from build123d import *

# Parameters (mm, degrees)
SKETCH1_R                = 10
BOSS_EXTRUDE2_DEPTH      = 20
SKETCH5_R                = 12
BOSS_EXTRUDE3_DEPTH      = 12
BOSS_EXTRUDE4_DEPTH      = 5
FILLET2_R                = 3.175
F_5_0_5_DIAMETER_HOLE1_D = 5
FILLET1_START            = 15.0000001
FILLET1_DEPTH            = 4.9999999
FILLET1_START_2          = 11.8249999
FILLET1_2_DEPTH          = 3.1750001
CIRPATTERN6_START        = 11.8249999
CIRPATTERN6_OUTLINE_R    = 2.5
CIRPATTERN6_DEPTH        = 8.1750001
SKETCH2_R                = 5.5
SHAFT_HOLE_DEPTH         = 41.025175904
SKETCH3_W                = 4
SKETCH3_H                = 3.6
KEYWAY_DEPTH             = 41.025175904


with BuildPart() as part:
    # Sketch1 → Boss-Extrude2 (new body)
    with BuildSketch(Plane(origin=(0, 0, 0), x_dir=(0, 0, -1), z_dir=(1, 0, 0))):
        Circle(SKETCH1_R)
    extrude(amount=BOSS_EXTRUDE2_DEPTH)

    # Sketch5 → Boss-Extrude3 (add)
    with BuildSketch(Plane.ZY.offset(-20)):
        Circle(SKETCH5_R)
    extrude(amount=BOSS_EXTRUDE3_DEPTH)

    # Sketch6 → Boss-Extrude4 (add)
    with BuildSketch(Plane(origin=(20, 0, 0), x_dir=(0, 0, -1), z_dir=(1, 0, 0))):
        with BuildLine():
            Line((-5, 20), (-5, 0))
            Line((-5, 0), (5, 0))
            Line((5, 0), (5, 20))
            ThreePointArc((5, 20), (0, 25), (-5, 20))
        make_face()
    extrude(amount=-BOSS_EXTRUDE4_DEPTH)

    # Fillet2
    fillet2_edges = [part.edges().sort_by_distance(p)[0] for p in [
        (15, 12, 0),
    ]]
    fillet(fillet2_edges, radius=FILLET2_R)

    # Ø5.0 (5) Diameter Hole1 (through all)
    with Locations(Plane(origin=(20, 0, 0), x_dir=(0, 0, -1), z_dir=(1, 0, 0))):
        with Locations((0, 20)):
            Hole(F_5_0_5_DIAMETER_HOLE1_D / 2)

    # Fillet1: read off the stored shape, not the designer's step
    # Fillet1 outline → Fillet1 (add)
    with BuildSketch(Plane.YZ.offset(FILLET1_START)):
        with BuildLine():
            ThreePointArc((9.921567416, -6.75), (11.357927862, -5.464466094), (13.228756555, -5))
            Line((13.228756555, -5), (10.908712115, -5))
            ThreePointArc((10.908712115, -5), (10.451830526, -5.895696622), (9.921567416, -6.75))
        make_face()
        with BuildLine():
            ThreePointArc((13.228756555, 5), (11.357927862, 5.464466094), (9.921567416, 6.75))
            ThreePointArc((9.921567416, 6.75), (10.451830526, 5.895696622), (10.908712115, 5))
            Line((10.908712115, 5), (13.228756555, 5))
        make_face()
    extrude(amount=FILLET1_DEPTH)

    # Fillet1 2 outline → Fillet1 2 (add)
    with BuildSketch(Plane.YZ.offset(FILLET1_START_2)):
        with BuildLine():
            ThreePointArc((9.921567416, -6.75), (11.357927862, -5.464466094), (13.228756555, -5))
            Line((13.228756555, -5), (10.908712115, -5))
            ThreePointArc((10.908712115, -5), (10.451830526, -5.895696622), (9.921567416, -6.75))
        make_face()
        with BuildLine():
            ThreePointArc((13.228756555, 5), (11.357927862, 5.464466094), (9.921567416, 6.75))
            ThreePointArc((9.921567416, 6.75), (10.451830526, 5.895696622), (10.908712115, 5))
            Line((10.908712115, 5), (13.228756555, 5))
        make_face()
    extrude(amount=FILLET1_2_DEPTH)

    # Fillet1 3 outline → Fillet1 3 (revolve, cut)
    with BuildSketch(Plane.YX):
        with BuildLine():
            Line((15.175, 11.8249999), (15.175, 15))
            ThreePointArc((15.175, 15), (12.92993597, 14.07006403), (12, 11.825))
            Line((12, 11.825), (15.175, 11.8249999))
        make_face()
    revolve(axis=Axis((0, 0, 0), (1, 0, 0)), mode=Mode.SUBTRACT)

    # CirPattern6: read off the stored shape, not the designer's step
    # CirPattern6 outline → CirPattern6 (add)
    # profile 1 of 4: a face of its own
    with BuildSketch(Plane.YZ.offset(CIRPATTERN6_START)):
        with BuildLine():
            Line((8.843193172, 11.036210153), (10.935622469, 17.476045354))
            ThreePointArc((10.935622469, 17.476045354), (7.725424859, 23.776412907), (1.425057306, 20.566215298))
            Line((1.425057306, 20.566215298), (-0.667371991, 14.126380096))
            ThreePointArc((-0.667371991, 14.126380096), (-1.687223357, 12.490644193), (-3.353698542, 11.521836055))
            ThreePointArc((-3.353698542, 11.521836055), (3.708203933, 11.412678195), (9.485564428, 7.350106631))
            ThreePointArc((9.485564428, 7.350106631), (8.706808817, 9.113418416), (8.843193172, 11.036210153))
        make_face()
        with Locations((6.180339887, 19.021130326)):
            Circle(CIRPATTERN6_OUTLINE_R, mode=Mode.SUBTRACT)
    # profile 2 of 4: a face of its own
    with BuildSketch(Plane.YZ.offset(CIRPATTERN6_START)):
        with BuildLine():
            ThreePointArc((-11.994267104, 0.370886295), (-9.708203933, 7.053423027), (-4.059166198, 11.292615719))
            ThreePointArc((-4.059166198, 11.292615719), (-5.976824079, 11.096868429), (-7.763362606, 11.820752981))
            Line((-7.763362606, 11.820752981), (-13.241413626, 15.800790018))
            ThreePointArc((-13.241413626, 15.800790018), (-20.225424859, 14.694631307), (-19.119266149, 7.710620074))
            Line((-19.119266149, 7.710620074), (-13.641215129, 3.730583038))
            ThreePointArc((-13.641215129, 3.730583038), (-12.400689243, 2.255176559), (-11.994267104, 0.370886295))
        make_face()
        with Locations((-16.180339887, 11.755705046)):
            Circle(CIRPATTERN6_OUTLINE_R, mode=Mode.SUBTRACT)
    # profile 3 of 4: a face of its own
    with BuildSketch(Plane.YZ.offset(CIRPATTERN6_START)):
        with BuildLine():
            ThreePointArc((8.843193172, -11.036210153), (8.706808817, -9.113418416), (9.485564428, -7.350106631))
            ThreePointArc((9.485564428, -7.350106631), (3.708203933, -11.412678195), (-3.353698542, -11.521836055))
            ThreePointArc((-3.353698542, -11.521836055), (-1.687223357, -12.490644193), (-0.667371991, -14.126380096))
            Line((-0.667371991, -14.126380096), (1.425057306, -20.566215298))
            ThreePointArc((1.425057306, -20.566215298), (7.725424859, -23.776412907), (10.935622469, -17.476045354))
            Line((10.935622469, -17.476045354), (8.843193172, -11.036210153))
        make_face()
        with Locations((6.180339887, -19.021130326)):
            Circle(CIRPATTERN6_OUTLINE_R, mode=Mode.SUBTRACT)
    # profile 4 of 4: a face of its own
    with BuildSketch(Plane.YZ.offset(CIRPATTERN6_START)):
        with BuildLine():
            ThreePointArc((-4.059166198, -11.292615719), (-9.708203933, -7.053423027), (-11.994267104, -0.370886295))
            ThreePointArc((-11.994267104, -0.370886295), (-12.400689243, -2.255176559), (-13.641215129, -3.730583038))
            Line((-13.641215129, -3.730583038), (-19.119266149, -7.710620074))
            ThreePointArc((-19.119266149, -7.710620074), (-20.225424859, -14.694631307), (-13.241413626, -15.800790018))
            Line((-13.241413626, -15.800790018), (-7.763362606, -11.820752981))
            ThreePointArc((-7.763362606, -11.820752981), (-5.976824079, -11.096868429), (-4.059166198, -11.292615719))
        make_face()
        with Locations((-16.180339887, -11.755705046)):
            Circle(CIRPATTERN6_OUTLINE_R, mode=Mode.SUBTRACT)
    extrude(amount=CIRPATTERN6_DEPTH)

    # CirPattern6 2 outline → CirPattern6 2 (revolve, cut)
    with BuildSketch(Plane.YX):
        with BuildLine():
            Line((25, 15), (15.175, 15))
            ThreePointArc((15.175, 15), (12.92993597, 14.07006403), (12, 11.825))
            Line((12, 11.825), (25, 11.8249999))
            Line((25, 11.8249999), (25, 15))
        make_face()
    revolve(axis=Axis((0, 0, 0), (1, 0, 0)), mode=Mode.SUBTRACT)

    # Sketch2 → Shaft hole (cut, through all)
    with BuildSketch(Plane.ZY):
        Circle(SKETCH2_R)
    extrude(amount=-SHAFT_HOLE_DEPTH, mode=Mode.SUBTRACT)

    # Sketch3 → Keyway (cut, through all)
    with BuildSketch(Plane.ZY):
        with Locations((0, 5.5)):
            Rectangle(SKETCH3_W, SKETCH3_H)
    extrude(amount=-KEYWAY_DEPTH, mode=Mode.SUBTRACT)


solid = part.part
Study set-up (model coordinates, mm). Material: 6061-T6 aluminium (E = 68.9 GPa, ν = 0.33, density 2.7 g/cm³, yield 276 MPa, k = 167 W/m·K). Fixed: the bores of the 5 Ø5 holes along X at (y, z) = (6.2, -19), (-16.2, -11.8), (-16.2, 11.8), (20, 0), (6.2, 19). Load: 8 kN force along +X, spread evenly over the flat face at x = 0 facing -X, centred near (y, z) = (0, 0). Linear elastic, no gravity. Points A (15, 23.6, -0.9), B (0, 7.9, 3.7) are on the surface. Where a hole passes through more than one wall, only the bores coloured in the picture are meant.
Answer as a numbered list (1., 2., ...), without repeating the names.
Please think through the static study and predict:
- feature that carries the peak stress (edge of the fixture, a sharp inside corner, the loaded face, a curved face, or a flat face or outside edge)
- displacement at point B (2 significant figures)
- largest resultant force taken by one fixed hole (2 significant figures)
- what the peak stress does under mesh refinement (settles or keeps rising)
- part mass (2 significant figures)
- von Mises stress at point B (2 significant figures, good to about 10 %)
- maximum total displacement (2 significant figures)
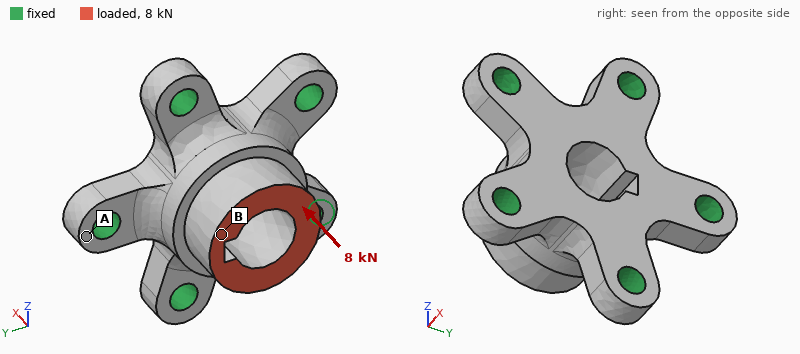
1. edge of the fixture
2. 26 µm
3. 1.9 kN
4. keeps rising
5. 23 g
6. 38 MPa
7. 27 µm
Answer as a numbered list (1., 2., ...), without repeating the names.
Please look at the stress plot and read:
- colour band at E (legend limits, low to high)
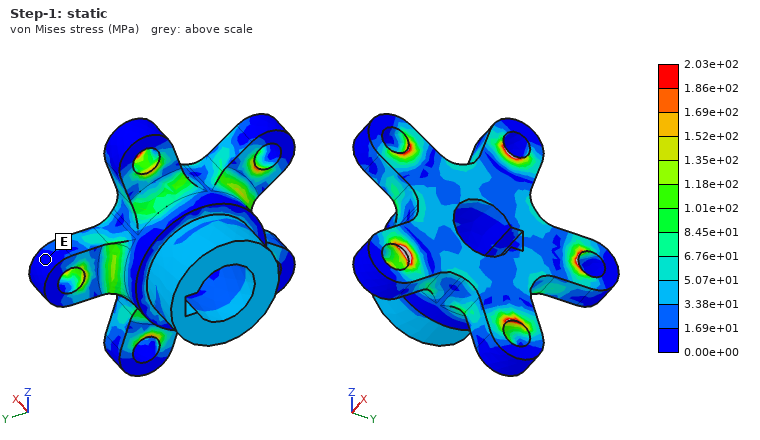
1. 0.00e+00 to 1.69e+01 MPa
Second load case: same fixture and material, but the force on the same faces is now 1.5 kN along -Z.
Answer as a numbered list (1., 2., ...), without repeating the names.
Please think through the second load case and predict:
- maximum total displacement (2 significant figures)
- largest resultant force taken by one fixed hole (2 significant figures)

1. 19 µm
2. 790 N
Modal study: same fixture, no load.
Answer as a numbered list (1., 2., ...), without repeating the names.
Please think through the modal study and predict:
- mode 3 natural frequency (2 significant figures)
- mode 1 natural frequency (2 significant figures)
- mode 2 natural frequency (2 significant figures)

1. 24 kHz
2. 24 kHz
3. 24 kHz
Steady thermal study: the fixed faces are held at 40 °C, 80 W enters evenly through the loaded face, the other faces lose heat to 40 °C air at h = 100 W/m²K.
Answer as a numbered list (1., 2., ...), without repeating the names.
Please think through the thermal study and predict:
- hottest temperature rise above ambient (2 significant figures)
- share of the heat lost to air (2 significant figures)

1. 43 K
2. 7.6 %
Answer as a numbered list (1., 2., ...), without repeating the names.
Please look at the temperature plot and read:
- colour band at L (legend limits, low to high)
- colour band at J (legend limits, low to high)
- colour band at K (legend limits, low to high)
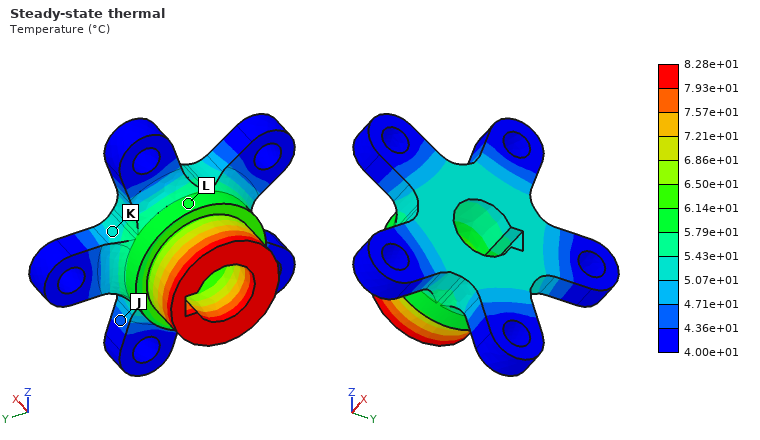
1. 5.79e+01 to 6.14e+01 °C
2. 4.36e+01 to 4.71e+01 °C
3. 5.07e+01 to 5.43e+01 °C
